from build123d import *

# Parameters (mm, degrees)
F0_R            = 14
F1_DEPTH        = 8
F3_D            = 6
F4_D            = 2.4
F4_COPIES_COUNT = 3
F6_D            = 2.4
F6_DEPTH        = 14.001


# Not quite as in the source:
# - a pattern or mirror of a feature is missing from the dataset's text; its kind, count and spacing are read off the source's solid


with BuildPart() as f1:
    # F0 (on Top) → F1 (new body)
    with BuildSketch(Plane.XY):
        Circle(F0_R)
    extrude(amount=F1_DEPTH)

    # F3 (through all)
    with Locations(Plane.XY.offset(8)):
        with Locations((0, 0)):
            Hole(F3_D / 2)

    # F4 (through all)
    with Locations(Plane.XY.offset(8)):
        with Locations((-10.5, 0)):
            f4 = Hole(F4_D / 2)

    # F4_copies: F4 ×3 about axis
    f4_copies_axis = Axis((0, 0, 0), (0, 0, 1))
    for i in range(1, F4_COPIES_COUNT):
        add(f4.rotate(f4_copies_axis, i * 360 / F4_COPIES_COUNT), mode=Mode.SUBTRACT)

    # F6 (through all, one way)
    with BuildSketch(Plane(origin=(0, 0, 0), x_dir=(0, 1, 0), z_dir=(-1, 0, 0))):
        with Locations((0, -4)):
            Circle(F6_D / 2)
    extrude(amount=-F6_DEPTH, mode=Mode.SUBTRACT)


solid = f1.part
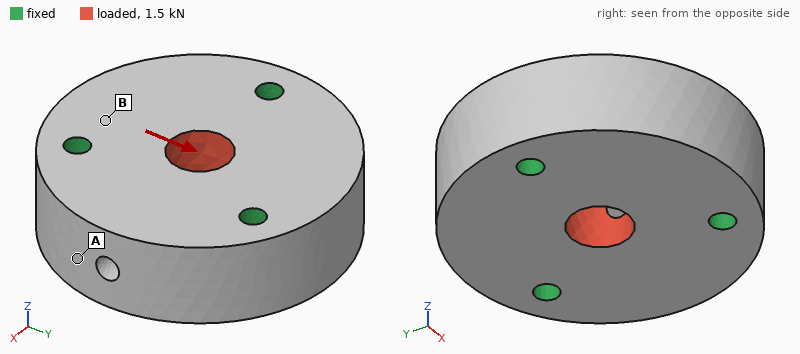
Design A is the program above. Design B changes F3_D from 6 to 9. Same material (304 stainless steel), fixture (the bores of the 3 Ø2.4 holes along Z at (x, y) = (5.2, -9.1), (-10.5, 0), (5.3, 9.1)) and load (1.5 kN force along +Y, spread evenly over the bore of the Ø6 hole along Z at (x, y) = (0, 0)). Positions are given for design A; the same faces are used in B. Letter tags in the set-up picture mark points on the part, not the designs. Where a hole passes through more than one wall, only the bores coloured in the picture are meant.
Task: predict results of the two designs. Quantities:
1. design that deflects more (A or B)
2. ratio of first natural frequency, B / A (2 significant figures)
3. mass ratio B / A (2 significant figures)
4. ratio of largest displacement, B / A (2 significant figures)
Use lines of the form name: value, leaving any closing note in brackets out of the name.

design that deflects more: A
ratio of first natural frequency, B / A: 0.99
mass ratio B / A: 0.94
ratio of largest displacement, B / A: 0.87
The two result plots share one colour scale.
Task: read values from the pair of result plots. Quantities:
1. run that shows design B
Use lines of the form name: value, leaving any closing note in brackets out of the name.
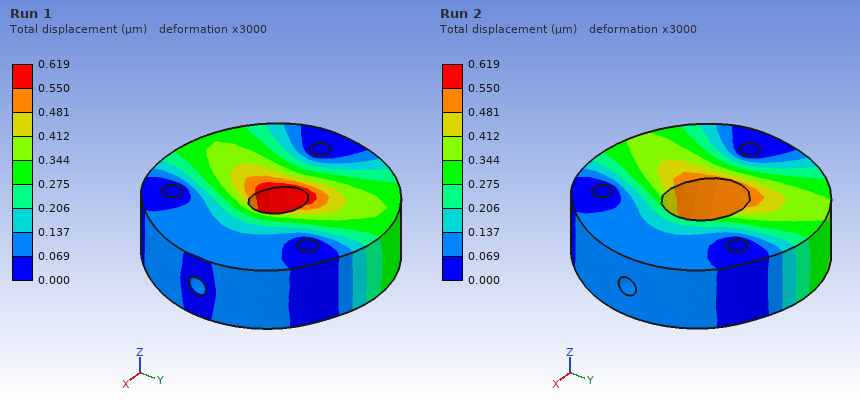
run that shows design B: Run 2
